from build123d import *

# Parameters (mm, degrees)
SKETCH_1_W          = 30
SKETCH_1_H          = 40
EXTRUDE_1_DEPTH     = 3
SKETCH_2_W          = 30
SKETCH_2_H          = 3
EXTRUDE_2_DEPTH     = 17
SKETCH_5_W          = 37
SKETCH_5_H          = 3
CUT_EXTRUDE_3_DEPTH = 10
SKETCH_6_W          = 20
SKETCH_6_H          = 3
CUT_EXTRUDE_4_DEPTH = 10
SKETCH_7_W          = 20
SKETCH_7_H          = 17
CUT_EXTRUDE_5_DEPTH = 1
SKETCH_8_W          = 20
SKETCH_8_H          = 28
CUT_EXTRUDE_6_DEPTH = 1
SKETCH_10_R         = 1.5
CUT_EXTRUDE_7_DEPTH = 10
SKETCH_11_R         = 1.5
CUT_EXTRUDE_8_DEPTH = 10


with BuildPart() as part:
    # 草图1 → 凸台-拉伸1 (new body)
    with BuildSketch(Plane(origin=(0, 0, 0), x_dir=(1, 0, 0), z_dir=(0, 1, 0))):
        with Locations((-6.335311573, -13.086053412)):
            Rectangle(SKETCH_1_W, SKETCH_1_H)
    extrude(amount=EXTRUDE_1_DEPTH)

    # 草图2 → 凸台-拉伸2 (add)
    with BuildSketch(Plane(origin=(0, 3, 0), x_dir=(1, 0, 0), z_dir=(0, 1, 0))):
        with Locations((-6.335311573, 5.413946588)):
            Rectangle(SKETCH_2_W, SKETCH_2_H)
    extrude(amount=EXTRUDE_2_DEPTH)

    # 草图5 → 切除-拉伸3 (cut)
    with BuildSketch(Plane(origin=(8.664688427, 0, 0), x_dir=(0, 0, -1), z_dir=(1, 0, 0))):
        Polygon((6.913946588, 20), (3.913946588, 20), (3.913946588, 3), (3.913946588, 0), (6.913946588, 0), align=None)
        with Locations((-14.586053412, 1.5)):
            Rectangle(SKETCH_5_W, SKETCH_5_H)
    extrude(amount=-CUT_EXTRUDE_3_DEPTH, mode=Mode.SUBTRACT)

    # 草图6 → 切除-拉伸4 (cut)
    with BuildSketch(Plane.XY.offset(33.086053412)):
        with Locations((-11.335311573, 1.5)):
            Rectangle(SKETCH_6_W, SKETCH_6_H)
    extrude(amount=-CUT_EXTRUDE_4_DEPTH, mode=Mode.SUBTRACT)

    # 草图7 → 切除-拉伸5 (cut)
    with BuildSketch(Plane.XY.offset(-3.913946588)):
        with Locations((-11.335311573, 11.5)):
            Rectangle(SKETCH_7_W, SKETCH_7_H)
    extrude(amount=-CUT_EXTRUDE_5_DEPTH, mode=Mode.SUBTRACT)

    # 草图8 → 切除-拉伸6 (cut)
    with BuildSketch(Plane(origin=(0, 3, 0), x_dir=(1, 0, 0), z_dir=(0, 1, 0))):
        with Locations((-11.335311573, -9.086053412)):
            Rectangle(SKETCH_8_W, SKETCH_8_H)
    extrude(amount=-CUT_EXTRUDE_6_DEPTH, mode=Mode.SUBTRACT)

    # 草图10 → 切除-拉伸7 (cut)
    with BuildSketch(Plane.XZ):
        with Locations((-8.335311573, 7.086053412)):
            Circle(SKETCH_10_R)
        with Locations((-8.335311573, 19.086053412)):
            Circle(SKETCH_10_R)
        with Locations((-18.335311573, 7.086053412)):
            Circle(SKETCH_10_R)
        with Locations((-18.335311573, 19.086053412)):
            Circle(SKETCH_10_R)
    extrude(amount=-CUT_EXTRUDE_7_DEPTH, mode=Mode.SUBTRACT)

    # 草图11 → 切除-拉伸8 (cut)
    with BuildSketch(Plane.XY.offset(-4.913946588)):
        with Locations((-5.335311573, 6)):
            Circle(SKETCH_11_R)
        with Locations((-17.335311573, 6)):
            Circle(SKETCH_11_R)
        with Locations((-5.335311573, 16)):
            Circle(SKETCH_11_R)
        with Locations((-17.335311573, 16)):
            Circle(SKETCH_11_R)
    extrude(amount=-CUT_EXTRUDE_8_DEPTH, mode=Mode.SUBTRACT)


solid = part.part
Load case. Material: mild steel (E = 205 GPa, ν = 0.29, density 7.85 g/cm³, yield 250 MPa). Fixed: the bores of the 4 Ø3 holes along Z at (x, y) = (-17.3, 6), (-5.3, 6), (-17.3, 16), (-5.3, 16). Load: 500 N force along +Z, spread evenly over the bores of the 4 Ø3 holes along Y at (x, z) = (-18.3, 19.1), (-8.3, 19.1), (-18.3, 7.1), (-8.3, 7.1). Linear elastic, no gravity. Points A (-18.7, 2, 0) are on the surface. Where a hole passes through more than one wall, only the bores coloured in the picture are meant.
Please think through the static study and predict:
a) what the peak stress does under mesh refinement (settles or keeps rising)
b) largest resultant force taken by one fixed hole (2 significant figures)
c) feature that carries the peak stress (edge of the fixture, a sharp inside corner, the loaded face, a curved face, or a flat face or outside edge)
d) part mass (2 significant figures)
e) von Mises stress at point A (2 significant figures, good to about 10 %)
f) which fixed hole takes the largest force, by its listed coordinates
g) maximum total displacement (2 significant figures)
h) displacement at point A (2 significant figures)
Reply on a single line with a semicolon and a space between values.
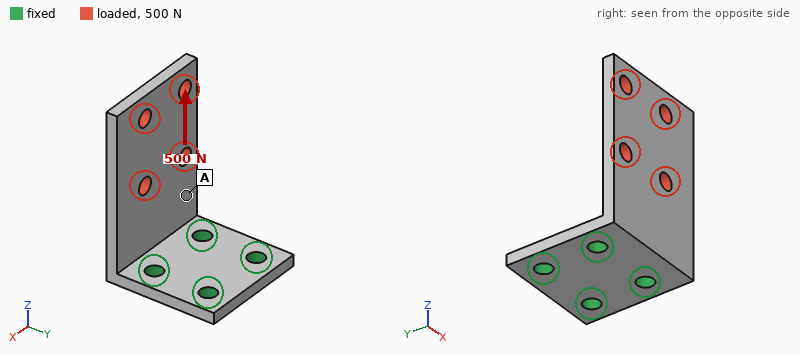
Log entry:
keeps rising; 340 N; edge of the fixture; 14 g; 24 MPa; (-17.3, 6); 54 µm; 13 µm
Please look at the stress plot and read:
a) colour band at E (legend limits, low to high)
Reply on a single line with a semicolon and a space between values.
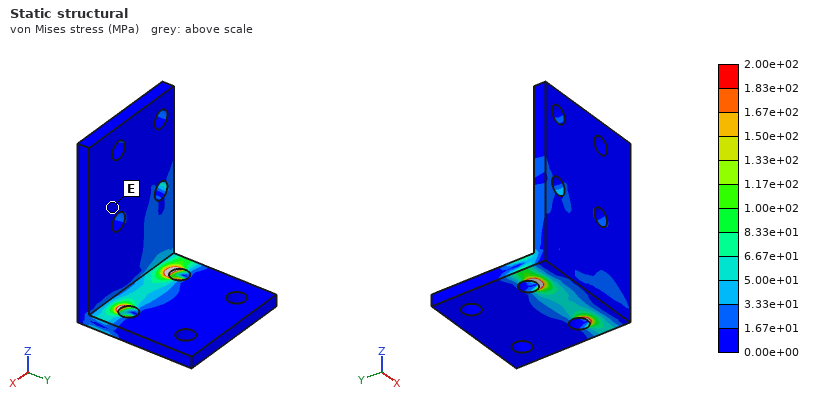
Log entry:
0.00e+00 to 1.67e+01 MPa
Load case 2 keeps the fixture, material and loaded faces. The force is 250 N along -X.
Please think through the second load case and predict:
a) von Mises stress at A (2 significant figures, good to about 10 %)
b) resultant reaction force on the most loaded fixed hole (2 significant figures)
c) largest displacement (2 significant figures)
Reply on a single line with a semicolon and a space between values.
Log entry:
45 MPa; 380 N; 35 µm
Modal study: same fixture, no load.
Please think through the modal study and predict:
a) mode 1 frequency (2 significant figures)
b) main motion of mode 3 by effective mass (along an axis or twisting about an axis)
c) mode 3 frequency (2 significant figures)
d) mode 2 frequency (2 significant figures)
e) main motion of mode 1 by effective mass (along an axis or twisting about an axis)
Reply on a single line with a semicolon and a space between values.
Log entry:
1700 Hz; along X; 7300 Hz; 5500 Hz; along Y
